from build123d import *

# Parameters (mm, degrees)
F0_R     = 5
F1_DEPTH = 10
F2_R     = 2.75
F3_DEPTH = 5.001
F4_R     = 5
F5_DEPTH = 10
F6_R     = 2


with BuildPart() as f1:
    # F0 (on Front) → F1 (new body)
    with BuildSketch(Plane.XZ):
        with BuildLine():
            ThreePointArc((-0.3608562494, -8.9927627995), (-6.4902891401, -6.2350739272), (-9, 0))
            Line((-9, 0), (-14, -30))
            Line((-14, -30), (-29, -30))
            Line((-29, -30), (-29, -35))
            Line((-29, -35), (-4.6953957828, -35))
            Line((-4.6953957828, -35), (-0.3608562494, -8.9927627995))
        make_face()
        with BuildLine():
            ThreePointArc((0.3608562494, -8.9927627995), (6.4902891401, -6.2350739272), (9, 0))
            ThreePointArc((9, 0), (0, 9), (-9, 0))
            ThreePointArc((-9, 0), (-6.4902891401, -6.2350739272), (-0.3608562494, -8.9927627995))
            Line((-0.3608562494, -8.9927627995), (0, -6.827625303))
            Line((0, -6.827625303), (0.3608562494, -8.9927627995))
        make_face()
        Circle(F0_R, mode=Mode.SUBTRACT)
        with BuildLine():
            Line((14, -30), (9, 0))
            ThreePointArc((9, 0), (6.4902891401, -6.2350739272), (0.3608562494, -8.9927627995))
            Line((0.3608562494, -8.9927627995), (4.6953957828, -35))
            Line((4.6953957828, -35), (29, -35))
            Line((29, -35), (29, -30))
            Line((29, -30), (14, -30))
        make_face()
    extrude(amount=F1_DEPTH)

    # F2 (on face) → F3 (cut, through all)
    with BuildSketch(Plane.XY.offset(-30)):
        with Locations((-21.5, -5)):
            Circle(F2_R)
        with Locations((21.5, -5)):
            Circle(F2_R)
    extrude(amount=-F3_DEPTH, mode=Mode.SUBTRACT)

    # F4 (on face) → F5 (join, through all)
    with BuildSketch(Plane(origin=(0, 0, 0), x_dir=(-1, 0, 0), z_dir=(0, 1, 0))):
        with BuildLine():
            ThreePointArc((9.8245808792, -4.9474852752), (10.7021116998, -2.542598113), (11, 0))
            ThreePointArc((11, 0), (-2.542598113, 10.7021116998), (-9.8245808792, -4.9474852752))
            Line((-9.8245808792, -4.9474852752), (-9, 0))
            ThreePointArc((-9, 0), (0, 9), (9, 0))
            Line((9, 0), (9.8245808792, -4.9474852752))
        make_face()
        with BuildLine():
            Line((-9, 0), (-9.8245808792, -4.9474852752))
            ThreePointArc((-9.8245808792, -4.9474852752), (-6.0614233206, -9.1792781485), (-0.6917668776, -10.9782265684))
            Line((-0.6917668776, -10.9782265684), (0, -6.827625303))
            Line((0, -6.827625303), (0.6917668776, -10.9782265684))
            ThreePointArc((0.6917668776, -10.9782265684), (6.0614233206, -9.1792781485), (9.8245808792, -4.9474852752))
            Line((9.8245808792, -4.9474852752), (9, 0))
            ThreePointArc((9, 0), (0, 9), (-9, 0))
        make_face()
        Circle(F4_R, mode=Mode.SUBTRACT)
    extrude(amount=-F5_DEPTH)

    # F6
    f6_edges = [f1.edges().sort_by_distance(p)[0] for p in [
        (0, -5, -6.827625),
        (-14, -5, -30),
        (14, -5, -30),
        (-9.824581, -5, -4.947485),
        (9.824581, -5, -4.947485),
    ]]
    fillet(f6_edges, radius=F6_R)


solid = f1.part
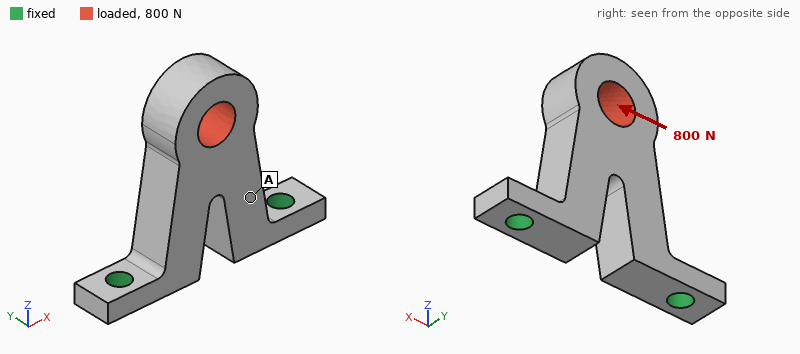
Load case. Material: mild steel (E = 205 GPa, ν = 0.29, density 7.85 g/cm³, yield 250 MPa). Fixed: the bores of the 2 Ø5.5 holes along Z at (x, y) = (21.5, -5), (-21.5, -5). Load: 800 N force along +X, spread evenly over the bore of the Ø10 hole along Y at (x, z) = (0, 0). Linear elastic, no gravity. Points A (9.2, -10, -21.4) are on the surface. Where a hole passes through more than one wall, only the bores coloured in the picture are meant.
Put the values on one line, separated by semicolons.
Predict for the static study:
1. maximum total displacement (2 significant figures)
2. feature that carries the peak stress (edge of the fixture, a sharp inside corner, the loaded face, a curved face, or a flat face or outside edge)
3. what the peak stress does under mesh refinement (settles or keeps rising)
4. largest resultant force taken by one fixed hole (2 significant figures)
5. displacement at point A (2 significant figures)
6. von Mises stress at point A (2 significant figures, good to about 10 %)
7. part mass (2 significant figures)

16 µm; edge of the fixture; keeps rising; 890 N; 3.3 µm; 16 MPa; 76 g
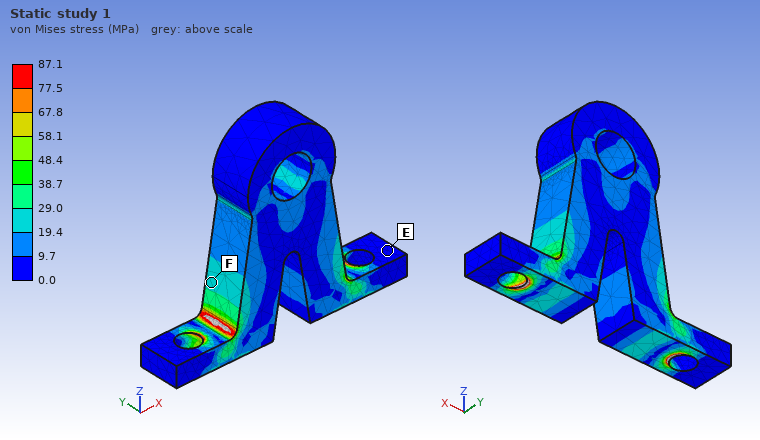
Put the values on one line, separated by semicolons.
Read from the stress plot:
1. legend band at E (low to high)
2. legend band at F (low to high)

0.0 to 9.7 MPa; 19.4 to 29.0 MPa
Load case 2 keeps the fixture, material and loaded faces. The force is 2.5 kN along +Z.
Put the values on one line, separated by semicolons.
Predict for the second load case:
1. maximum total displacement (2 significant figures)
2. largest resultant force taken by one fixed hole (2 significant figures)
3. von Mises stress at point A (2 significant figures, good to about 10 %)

8.9 µm; 1.4 kN; 23 MPa
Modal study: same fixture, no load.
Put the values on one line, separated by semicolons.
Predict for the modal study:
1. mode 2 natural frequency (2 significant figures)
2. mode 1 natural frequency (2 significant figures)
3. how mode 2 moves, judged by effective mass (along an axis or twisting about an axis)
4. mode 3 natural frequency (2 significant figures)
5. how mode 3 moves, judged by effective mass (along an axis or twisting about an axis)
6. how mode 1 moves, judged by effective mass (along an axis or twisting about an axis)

7600 Hz; 2200 Hz; along X; 12 kHz; along Z; along Y
